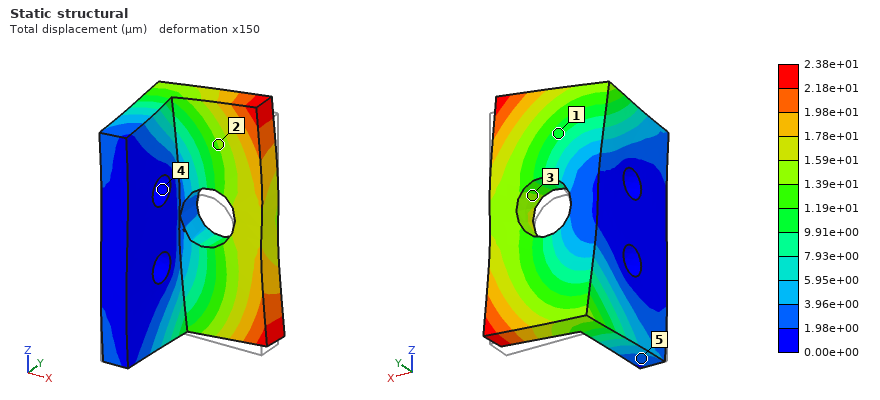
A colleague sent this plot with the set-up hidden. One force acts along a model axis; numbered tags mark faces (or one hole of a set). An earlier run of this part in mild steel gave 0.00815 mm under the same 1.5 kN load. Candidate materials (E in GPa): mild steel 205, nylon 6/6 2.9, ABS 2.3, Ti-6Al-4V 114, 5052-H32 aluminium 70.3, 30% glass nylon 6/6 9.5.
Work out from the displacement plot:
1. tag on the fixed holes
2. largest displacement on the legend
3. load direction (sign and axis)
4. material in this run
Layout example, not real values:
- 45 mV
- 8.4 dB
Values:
- 4
- 2.38e+01 µm
- +Z
- 5052-H32 aluminium
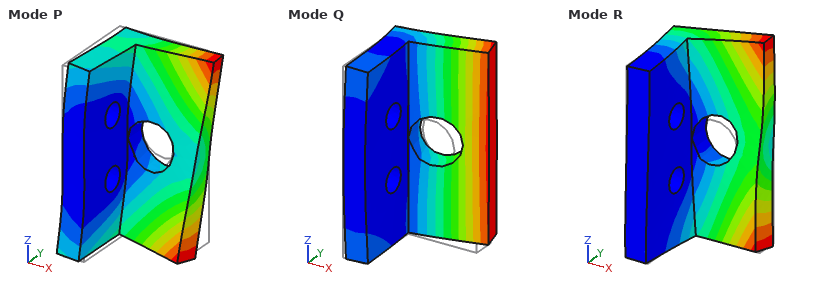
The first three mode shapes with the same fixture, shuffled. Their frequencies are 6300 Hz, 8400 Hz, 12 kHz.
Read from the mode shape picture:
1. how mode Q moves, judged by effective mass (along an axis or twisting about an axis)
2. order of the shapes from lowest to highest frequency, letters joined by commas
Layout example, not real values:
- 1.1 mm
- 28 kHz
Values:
- along Y
- Q, R, P
